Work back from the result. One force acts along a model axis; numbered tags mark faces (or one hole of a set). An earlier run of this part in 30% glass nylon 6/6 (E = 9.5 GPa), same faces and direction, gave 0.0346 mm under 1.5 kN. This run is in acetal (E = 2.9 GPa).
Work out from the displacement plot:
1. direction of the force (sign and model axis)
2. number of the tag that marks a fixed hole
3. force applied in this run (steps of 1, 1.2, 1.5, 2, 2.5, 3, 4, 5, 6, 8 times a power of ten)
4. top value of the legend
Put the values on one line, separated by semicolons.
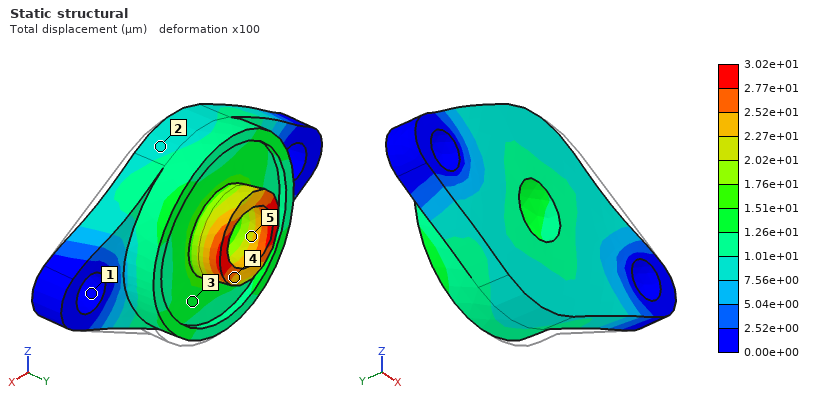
-X; 1; 400 N; 3.02e+01 µm
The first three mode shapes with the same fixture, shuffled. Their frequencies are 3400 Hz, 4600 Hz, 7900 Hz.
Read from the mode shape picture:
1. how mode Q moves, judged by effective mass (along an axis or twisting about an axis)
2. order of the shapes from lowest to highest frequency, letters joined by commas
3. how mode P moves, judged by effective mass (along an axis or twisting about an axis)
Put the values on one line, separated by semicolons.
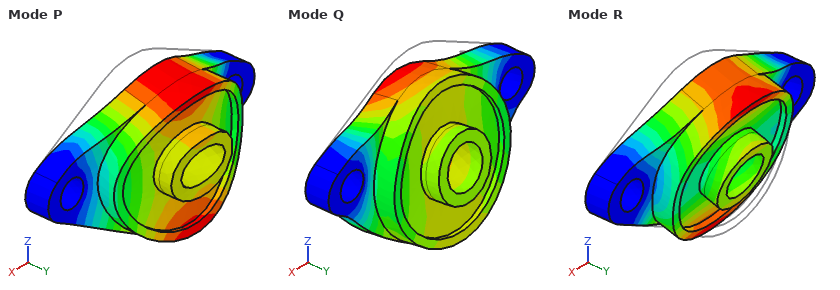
along Z; R, P, Q; along Y
